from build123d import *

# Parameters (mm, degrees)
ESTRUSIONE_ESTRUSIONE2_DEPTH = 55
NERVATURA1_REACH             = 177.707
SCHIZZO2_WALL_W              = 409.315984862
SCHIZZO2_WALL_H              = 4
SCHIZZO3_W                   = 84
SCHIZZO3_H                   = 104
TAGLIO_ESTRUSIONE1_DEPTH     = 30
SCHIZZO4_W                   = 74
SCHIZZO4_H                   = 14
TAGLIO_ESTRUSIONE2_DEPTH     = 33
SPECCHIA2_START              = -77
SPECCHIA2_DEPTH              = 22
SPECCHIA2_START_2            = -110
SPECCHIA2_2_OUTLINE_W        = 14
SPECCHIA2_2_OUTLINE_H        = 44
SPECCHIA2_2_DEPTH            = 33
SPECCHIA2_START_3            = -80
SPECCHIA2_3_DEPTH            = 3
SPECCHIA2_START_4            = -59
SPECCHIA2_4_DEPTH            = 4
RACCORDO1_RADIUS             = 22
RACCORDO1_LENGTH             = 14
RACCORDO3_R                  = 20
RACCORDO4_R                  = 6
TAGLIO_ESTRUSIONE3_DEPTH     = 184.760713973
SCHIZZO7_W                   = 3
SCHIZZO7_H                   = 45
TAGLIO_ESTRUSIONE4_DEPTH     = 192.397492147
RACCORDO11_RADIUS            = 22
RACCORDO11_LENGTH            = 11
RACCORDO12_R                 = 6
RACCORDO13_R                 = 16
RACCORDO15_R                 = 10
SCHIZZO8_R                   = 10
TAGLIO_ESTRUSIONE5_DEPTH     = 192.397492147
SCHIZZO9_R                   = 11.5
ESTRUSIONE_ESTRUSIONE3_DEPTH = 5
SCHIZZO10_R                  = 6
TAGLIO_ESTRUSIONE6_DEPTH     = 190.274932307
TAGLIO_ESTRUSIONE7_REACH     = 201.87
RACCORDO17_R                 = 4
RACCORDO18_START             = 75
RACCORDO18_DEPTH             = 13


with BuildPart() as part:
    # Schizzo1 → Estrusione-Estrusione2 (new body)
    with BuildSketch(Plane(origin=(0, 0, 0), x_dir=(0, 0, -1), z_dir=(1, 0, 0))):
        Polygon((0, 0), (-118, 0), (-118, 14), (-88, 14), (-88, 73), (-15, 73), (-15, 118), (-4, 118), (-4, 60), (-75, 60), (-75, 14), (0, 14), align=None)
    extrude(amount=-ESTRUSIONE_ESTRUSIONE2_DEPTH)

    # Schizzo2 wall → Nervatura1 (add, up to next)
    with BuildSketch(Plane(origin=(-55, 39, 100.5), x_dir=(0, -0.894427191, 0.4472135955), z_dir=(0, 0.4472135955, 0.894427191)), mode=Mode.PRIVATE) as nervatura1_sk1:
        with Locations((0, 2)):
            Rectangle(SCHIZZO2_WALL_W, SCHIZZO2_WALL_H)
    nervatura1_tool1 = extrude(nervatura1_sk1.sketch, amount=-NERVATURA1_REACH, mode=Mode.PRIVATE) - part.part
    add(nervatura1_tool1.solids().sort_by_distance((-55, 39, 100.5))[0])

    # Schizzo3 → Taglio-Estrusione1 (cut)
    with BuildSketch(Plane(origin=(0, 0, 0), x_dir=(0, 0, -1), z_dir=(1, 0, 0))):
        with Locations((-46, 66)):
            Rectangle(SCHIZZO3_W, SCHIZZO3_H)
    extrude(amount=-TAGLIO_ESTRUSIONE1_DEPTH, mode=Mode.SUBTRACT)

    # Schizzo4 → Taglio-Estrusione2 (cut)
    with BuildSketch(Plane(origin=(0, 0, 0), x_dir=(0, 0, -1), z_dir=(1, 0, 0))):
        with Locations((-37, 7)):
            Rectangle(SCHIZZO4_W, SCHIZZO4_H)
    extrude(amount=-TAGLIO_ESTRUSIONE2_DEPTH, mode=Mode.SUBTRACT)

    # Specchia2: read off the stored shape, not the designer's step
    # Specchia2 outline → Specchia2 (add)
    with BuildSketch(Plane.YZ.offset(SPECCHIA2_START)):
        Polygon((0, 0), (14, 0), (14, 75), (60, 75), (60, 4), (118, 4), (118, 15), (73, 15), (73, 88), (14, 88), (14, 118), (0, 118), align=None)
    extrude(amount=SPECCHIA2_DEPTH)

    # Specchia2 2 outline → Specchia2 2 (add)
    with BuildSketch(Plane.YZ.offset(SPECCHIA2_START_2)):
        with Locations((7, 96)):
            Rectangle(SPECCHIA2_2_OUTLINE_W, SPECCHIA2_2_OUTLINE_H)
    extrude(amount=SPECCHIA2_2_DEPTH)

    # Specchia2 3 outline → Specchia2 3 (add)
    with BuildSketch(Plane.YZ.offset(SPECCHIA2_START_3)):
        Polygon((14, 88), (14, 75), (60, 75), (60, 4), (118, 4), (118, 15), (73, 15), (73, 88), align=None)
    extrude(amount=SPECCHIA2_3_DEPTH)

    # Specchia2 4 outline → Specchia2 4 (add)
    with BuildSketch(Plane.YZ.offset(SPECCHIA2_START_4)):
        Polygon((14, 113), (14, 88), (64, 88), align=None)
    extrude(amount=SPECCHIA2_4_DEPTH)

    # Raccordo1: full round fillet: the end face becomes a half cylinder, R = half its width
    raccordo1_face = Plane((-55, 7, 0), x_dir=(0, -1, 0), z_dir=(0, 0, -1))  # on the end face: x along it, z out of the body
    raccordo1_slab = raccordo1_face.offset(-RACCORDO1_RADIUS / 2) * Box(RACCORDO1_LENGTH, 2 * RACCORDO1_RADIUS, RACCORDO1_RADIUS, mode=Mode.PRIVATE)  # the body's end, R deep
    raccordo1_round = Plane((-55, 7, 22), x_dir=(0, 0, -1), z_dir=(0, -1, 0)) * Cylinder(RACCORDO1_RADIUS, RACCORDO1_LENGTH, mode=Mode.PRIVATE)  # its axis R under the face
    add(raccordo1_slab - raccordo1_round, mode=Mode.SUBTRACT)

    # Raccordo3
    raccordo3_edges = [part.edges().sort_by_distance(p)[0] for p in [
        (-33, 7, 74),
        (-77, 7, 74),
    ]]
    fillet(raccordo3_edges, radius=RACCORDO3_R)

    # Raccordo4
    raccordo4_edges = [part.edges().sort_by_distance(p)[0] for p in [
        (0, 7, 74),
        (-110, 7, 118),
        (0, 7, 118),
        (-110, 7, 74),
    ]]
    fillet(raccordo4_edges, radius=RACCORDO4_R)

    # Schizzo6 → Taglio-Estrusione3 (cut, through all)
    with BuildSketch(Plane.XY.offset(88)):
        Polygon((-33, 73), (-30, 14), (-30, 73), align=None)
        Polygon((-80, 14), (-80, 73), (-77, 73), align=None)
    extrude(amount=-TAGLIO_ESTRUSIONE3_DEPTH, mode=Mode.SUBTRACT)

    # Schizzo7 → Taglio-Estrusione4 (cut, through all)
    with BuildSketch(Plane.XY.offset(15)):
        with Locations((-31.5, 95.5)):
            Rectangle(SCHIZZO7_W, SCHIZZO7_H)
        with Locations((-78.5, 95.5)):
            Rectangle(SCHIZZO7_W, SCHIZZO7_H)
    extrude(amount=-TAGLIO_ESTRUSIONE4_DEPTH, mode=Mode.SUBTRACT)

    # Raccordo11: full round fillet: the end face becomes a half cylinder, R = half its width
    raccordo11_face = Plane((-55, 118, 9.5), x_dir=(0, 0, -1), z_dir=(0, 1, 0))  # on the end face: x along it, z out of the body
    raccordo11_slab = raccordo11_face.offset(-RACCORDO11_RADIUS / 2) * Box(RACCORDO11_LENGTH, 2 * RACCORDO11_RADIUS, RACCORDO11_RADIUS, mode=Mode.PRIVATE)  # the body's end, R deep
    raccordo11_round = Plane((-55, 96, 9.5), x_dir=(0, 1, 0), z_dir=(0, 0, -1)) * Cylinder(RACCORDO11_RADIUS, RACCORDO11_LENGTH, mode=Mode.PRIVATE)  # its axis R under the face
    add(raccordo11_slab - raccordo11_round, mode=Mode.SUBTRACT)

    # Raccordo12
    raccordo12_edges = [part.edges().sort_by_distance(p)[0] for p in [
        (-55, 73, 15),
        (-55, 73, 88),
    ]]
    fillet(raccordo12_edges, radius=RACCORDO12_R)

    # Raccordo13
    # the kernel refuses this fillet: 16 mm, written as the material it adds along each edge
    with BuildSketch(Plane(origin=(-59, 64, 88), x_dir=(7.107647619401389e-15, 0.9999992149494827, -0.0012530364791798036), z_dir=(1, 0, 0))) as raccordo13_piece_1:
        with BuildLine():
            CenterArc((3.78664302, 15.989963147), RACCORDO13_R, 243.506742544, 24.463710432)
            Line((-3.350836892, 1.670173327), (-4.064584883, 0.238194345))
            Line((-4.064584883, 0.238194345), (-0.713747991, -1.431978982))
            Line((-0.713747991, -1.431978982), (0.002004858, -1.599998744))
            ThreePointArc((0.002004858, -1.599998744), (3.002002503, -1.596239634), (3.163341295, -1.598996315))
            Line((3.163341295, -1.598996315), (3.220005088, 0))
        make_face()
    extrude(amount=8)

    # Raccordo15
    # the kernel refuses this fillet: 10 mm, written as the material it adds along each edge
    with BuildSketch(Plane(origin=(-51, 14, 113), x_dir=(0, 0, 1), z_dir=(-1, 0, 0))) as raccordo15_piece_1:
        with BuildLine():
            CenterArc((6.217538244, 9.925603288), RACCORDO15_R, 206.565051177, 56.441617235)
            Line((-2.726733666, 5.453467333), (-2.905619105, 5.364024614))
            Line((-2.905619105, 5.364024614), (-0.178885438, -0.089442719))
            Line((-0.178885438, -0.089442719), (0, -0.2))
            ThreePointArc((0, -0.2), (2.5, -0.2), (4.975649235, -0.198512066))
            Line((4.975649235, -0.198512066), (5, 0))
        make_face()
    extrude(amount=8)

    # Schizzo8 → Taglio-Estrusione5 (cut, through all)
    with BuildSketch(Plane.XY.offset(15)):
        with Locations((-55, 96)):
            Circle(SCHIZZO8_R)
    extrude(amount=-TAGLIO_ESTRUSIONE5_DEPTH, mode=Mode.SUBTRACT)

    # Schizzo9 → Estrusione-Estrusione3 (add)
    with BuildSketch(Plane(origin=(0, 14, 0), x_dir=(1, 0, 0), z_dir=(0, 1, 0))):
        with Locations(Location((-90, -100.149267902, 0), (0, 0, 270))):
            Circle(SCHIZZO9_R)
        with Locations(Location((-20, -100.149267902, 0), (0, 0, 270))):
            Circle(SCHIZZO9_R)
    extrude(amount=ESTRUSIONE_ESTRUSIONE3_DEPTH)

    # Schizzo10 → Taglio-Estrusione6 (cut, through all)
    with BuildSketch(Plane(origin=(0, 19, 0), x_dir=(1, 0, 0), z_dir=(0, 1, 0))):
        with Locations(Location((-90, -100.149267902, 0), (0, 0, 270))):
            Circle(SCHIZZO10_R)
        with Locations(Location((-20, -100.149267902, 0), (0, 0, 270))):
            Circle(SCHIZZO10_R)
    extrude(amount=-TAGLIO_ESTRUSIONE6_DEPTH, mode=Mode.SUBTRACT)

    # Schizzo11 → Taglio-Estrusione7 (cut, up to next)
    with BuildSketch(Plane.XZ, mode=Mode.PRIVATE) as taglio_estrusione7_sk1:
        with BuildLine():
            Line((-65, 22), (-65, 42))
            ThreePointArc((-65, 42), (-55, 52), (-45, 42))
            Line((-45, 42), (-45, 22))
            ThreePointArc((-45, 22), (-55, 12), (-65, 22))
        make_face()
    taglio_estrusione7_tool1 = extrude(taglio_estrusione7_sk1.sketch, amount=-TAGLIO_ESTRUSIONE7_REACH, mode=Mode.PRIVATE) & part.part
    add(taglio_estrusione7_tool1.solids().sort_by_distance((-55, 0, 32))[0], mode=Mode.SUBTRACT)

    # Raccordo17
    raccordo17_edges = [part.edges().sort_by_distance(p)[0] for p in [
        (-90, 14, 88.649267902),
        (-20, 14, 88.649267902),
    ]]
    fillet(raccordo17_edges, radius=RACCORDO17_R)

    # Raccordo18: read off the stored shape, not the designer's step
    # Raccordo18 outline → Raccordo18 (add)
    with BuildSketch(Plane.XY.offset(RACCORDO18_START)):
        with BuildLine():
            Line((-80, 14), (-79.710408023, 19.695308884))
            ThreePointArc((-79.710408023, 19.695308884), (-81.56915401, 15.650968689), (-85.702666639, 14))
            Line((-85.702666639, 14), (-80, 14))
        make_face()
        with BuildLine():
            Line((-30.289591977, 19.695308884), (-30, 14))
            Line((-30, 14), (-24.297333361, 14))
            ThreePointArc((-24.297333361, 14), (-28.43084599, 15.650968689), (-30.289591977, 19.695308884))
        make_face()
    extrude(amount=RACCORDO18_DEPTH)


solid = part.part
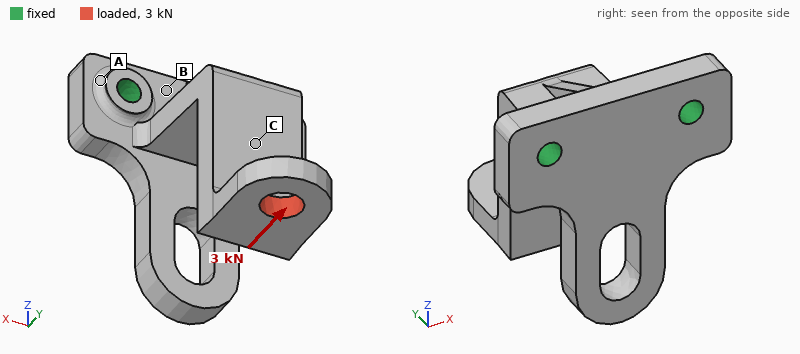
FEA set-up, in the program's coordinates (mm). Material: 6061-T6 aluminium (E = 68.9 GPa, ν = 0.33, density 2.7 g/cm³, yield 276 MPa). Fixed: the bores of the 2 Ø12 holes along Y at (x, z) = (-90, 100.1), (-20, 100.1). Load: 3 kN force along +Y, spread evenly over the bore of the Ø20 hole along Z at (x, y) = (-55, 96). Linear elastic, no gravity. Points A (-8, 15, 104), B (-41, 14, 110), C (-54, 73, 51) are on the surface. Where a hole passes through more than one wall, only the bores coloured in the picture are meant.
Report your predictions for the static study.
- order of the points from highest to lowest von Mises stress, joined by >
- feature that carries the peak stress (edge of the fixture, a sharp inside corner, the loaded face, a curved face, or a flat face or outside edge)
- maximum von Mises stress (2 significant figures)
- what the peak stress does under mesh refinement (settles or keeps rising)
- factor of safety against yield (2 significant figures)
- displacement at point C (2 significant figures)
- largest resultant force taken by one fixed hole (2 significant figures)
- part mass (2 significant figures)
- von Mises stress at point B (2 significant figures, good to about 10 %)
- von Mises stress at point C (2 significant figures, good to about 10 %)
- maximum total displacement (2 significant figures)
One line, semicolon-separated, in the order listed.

C > B > A; a curved face; 230 MPa; settles; 1.2; 0.70 mm; 1.7 kN; 540 g; 34 MPa; 93 MPa; 2.2 mm
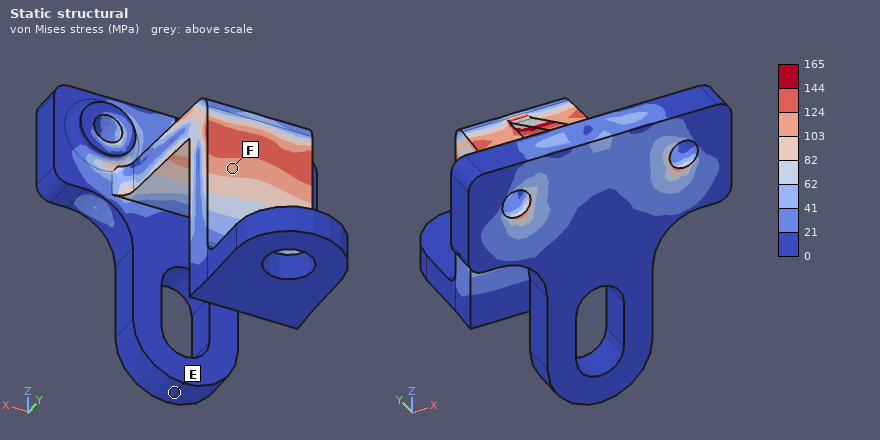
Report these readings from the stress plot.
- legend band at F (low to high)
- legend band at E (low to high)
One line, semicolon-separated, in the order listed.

103 to 124 MPa; 0 to 21 MPa
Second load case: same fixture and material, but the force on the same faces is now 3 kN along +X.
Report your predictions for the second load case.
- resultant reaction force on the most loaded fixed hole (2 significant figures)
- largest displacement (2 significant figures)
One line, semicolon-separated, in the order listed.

6.1 kN; 1.2 mm
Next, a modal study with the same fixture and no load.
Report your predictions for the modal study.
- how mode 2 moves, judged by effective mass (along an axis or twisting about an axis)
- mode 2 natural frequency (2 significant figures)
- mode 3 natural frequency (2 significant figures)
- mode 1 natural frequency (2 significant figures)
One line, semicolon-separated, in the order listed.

along X; 950 Hz; 1700 Hz; 660 Hz
